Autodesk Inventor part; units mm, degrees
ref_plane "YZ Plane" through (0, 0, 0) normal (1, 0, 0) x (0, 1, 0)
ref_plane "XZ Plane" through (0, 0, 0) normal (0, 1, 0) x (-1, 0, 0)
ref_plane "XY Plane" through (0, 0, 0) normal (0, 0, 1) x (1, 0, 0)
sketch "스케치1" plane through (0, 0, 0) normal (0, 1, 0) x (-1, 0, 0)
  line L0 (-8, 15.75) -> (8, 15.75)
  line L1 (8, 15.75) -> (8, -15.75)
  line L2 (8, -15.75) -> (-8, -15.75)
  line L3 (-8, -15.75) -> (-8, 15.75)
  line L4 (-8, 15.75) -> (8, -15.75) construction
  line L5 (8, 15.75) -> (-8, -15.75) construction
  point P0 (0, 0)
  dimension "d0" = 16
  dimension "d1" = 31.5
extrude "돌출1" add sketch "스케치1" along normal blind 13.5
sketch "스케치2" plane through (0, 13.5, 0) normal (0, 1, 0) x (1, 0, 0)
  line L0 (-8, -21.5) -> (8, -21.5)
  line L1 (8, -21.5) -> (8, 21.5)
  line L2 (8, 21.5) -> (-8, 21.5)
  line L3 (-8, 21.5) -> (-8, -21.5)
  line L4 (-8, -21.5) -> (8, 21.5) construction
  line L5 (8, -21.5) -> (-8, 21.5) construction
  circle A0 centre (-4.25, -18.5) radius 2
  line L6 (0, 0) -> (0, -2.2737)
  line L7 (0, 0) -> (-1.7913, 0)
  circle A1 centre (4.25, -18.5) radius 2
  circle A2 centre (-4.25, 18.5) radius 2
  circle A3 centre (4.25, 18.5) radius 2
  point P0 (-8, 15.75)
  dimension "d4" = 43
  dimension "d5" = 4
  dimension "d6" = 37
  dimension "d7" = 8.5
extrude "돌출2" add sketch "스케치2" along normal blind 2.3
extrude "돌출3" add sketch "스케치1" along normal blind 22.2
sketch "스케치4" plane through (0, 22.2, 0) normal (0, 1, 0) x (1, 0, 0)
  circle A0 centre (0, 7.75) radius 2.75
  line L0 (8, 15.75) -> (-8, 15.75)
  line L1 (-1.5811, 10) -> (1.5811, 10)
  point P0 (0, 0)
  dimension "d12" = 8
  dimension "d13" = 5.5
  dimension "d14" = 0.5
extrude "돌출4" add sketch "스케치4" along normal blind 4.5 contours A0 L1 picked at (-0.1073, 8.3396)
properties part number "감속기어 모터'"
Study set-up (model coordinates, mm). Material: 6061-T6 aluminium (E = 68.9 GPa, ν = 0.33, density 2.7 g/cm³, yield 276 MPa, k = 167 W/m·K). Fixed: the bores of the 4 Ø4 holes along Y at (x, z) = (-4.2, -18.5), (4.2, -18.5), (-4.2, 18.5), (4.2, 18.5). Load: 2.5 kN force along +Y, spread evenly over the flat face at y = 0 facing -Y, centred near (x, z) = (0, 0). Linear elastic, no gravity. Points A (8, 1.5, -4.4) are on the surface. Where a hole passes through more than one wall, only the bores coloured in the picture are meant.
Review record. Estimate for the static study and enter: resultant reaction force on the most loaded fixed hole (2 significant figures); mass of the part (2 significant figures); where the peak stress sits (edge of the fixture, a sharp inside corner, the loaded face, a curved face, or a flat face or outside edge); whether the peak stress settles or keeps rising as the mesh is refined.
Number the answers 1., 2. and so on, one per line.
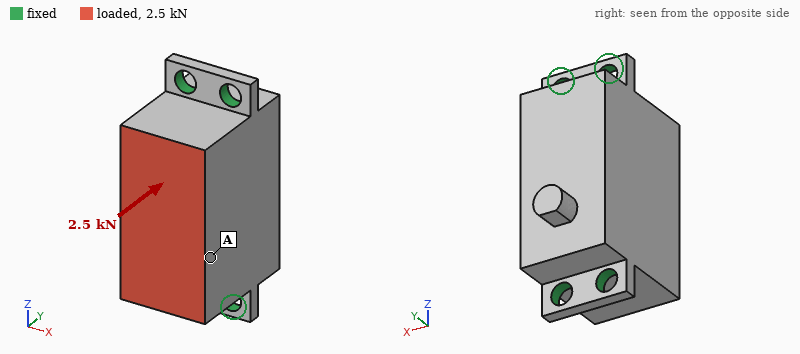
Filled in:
1. 630 N
2. 31 g
3. edge of the fixture
4. keeps rising
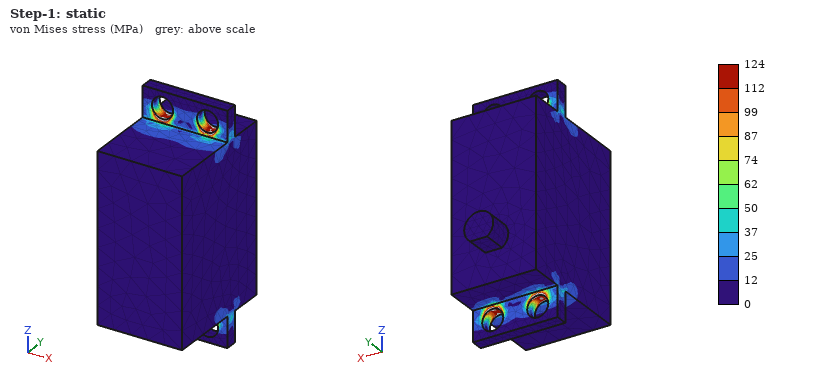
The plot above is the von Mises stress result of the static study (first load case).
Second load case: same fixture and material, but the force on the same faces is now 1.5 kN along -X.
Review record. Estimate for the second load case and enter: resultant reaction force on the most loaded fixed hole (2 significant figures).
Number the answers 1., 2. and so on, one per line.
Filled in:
1. 1.2 kN
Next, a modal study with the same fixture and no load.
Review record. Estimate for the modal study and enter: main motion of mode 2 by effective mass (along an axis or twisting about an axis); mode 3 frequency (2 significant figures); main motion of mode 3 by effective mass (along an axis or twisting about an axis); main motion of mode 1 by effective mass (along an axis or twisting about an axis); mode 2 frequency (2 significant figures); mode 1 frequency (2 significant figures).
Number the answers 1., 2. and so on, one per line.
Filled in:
1. along Y
2. 21 kHz
3. along X
4. along X
5. 19 kHz
6. 11 kHz
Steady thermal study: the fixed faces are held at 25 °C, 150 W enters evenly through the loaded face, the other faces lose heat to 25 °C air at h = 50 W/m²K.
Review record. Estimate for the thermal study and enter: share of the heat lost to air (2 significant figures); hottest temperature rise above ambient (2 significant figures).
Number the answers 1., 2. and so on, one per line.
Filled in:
1. 3.8 %
2. 64 K
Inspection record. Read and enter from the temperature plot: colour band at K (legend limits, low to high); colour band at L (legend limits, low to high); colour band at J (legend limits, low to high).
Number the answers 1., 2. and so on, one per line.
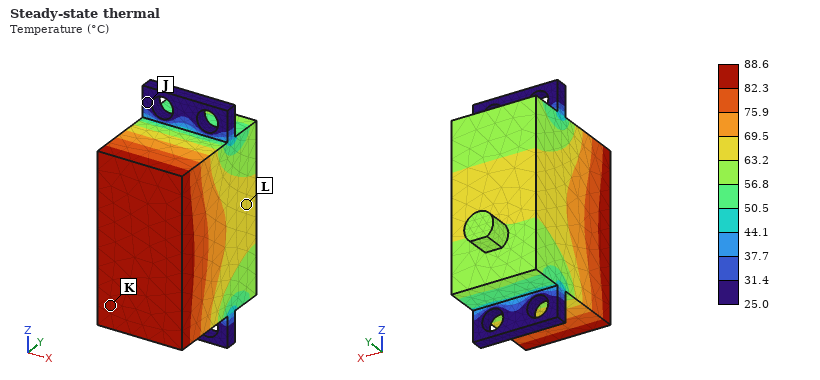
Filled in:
1. 82.3 to 88.6 °C
2. 63.2 to 69.5 °C
3. 25.0 to 31.4 °C
